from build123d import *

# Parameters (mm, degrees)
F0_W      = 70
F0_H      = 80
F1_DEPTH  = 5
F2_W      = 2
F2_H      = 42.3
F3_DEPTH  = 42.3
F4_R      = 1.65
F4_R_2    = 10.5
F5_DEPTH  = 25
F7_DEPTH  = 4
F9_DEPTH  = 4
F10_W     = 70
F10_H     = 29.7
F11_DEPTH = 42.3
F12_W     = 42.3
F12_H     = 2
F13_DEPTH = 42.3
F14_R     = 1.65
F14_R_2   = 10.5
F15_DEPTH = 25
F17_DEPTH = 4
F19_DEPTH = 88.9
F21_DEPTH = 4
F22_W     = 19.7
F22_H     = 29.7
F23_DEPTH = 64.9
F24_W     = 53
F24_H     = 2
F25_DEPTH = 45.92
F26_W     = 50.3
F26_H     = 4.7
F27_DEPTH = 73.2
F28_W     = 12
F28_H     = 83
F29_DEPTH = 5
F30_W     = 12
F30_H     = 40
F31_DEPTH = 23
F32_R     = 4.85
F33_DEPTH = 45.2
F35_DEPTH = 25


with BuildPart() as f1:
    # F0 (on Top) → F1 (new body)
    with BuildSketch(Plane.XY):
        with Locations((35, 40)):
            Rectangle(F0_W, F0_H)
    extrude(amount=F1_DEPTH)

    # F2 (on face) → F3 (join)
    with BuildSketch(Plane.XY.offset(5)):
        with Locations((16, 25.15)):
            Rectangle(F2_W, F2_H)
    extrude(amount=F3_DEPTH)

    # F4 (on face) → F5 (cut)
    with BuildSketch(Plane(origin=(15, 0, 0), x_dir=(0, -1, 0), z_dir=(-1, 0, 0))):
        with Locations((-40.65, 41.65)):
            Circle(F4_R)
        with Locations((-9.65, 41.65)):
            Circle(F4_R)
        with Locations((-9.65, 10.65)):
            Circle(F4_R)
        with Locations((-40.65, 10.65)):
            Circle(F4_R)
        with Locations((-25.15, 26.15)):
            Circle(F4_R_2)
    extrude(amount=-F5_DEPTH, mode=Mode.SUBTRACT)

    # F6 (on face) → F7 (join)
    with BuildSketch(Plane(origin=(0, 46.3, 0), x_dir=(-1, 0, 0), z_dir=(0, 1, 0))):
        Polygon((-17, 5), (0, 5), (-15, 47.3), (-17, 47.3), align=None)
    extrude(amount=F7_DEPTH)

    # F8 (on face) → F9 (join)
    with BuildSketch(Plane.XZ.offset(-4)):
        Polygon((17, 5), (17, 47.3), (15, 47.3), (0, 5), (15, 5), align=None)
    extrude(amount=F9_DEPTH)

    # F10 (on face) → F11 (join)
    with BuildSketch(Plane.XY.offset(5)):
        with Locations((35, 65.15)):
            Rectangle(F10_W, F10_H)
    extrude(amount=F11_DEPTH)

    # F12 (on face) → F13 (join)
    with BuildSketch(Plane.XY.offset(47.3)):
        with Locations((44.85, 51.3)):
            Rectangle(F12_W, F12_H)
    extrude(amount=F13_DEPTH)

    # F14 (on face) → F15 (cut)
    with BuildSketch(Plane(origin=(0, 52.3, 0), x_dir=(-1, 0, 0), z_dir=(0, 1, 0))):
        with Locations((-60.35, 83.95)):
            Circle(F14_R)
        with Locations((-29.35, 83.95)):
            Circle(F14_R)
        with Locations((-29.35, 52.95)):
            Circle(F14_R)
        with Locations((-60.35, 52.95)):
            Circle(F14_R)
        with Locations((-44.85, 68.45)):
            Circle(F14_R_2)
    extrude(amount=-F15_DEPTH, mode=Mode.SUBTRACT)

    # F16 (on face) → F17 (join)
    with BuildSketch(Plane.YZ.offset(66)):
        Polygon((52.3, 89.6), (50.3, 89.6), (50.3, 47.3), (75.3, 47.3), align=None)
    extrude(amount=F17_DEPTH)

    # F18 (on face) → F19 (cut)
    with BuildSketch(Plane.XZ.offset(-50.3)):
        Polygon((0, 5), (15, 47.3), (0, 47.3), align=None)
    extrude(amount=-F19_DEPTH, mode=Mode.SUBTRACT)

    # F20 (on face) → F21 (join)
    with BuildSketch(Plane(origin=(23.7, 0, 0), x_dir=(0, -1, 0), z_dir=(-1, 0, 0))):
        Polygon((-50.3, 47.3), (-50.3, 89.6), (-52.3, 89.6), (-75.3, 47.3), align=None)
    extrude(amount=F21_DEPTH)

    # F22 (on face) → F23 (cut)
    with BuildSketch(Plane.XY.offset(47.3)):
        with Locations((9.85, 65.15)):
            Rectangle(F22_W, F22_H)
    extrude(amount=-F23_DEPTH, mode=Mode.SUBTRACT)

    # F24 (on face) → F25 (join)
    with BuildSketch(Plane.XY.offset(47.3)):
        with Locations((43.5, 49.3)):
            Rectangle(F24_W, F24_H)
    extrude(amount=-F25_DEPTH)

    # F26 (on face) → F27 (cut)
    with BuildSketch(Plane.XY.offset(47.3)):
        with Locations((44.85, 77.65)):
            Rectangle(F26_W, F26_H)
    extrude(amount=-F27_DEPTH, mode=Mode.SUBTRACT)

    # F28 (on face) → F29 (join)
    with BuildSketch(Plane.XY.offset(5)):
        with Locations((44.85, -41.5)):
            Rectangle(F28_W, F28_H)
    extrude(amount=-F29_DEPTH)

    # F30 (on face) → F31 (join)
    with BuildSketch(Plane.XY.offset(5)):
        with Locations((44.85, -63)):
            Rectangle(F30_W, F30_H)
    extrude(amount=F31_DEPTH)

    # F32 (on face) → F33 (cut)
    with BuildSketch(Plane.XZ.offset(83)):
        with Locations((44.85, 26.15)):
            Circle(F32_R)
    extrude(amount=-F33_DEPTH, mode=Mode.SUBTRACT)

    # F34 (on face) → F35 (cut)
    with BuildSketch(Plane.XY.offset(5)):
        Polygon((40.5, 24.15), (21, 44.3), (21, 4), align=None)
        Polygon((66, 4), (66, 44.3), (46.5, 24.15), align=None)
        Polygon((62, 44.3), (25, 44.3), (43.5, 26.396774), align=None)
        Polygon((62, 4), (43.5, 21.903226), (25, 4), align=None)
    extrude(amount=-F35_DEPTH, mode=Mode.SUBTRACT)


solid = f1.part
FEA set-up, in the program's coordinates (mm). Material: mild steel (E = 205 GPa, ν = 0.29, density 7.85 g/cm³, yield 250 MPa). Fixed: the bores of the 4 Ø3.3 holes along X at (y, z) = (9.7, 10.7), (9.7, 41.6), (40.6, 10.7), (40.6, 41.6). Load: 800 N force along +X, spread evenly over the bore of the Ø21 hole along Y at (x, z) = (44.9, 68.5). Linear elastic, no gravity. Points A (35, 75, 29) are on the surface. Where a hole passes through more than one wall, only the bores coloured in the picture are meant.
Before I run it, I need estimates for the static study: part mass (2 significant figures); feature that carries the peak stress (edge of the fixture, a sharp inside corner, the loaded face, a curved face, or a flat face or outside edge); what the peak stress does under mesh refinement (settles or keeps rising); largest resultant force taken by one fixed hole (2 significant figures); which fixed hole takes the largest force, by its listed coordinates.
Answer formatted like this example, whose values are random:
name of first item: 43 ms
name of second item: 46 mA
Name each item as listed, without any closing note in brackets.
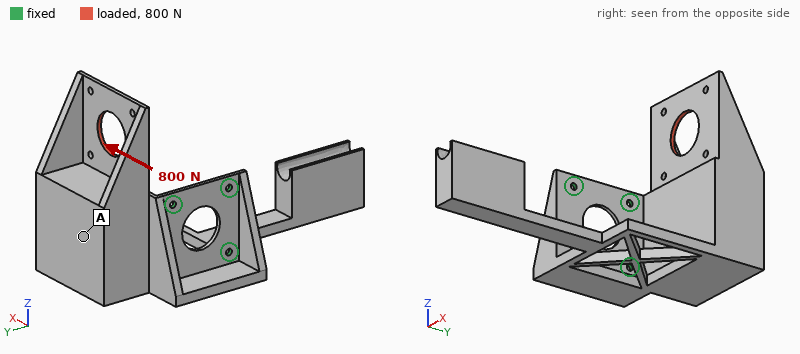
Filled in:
part mass: 800 g
feature that carries the peak stress: edge of the fixture
what the peak stress does under mesh refinement: keeps rising
largest resultant force taken by one fixed hole: 1.4 kN
which fixed hole takes the largest force, by its listed coordinates: (40.6, 41.6)
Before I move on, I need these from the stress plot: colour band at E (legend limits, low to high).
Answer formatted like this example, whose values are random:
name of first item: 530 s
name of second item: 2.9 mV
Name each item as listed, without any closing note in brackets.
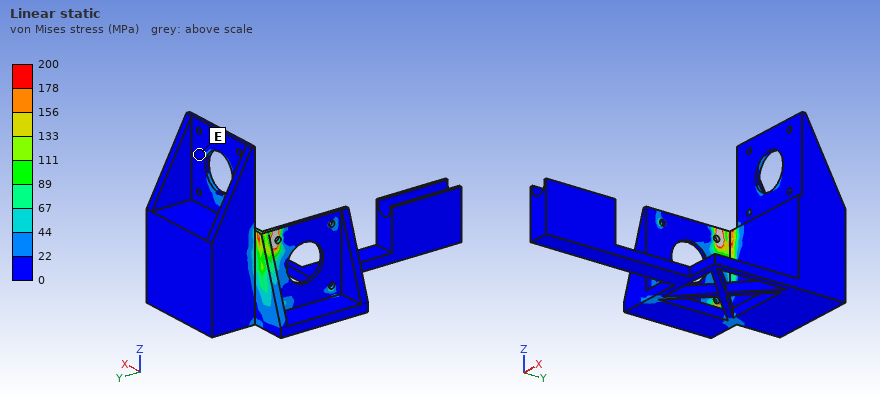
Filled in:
colour band at E: 0 to 22 MPa
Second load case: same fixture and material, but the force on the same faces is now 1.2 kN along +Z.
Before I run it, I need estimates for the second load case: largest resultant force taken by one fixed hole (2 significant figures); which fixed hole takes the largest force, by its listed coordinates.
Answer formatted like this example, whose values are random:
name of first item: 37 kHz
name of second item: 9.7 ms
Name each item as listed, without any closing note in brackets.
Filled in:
largest resultant force taken by one fixed hole: 1.4 kN
which fixed hole takes the largest force, by its listed coordinates: (40.6, 10.7)
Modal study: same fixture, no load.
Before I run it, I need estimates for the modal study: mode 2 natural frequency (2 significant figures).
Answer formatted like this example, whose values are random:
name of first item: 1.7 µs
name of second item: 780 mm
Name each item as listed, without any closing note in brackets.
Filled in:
mode 2 natural frequency: 340 Hz
